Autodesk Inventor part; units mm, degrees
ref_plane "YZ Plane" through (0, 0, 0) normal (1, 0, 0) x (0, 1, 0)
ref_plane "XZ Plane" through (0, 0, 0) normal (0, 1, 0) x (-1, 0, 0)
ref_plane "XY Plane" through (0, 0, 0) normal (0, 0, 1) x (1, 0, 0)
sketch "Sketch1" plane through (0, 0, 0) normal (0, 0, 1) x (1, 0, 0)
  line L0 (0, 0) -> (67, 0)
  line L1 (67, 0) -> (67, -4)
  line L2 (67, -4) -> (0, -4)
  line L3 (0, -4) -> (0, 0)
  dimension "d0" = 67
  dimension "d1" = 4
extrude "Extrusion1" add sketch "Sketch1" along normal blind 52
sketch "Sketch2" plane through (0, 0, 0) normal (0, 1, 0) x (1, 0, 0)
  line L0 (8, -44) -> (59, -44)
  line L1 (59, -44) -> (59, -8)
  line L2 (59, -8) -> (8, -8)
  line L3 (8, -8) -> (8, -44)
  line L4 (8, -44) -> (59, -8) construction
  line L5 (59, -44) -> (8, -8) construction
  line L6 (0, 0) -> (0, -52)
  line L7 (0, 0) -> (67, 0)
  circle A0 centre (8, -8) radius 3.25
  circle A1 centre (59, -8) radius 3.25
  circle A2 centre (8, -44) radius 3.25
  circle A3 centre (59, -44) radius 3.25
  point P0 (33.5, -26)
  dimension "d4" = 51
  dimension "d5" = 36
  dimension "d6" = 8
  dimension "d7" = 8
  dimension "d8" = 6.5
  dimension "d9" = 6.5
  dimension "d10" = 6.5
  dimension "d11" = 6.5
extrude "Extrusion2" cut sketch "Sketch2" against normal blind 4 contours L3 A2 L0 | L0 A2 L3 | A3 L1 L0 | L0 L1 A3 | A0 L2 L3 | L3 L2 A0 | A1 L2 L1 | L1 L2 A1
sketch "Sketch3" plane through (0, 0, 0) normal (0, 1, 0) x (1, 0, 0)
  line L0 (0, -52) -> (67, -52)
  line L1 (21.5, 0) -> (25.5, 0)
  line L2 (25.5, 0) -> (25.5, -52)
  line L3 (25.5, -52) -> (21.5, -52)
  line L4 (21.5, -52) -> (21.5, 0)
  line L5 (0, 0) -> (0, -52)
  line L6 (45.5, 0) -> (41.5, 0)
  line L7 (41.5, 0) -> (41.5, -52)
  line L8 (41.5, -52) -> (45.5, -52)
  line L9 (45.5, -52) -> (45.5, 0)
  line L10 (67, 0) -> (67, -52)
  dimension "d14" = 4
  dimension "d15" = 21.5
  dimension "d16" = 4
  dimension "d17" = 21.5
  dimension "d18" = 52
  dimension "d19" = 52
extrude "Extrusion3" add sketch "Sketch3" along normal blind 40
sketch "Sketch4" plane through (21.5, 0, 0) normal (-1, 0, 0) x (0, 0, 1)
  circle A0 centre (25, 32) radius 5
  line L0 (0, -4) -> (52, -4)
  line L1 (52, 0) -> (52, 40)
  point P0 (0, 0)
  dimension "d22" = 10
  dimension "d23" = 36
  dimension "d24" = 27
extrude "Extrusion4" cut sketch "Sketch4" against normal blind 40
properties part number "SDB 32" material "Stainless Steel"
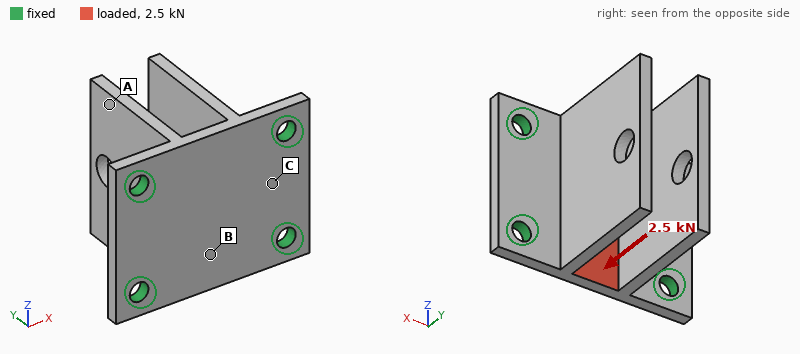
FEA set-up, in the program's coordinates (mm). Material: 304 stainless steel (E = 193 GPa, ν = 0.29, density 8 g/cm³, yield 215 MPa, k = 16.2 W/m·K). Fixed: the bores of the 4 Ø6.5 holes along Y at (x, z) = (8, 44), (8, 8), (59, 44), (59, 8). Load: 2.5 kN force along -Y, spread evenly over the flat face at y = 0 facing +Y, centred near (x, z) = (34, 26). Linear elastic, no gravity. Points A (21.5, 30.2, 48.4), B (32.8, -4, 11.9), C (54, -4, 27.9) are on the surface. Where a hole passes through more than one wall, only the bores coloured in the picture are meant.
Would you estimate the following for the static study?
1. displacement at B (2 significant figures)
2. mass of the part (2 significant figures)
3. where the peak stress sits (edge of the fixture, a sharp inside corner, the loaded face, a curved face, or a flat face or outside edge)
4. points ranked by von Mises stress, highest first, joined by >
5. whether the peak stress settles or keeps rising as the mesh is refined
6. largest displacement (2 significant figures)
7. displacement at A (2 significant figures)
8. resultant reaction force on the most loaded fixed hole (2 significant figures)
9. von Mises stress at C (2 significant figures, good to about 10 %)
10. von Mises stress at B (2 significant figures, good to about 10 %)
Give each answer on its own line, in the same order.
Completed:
28 µm
240 g
edge of the fixture
B > C > A
keeps rising
68 µm
52 µm
630 N
26 MPa
72 MPa
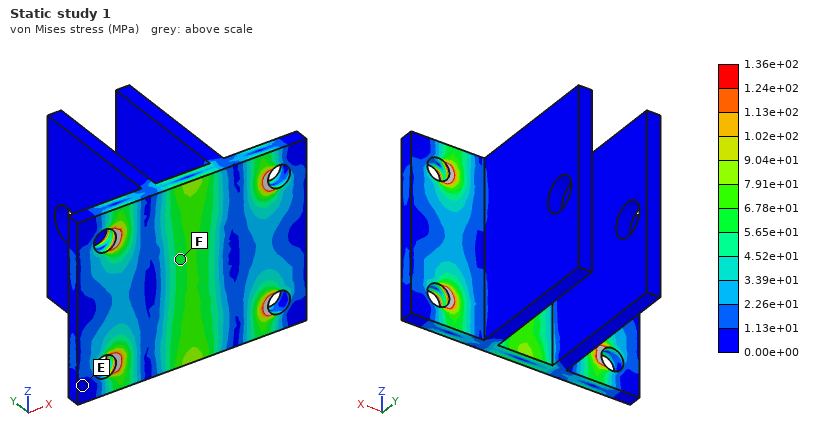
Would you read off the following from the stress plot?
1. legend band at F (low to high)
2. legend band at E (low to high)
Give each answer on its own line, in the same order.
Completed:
5.65e+01 to 6.78e+01 MPa
0.00e+00 to 1.13e+01 MPa
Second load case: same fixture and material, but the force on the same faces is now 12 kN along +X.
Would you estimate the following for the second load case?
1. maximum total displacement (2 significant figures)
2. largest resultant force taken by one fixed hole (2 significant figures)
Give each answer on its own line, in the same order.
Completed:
5.7 µm
3.1 kN
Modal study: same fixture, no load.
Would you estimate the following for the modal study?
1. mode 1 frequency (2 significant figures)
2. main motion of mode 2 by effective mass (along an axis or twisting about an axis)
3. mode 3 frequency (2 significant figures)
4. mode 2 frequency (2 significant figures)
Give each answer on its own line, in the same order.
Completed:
1600 Hz
along X
3200 Hz
1900 Hz
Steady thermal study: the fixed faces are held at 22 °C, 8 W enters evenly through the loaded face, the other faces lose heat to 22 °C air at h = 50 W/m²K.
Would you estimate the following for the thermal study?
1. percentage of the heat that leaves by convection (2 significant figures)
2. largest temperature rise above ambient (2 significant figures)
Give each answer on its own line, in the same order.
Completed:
54 %
17 K
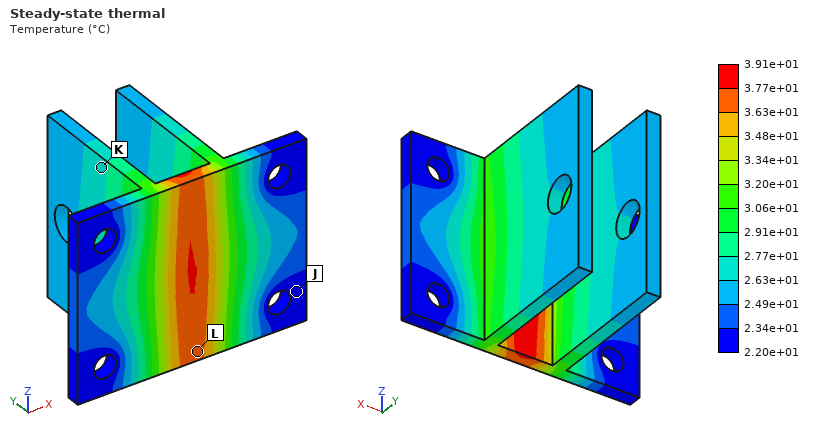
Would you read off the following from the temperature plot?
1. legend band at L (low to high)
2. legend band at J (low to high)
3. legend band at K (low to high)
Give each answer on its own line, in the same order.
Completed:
3.63e+01 to 3.77e+01 °C
2.20e+01 to 2.34e+01 °C
2.63e+01 to 2.77e+01 °C
